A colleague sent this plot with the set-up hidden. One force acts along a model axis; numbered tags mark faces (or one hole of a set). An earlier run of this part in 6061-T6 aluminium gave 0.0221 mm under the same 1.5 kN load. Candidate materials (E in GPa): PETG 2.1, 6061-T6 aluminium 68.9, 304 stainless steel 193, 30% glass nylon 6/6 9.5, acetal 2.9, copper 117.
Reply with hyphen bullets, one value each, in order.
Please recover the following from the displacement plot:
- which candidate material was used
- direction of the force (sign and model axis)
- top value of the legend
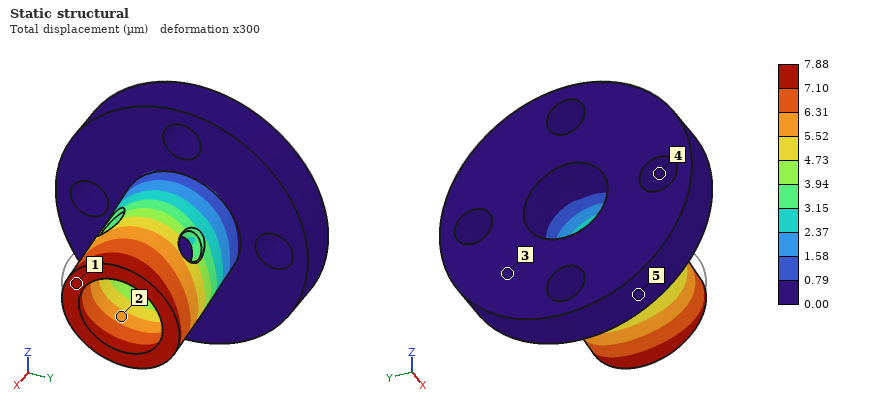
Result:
- 304 stainless steel
- -Z
- 7.88 µm
